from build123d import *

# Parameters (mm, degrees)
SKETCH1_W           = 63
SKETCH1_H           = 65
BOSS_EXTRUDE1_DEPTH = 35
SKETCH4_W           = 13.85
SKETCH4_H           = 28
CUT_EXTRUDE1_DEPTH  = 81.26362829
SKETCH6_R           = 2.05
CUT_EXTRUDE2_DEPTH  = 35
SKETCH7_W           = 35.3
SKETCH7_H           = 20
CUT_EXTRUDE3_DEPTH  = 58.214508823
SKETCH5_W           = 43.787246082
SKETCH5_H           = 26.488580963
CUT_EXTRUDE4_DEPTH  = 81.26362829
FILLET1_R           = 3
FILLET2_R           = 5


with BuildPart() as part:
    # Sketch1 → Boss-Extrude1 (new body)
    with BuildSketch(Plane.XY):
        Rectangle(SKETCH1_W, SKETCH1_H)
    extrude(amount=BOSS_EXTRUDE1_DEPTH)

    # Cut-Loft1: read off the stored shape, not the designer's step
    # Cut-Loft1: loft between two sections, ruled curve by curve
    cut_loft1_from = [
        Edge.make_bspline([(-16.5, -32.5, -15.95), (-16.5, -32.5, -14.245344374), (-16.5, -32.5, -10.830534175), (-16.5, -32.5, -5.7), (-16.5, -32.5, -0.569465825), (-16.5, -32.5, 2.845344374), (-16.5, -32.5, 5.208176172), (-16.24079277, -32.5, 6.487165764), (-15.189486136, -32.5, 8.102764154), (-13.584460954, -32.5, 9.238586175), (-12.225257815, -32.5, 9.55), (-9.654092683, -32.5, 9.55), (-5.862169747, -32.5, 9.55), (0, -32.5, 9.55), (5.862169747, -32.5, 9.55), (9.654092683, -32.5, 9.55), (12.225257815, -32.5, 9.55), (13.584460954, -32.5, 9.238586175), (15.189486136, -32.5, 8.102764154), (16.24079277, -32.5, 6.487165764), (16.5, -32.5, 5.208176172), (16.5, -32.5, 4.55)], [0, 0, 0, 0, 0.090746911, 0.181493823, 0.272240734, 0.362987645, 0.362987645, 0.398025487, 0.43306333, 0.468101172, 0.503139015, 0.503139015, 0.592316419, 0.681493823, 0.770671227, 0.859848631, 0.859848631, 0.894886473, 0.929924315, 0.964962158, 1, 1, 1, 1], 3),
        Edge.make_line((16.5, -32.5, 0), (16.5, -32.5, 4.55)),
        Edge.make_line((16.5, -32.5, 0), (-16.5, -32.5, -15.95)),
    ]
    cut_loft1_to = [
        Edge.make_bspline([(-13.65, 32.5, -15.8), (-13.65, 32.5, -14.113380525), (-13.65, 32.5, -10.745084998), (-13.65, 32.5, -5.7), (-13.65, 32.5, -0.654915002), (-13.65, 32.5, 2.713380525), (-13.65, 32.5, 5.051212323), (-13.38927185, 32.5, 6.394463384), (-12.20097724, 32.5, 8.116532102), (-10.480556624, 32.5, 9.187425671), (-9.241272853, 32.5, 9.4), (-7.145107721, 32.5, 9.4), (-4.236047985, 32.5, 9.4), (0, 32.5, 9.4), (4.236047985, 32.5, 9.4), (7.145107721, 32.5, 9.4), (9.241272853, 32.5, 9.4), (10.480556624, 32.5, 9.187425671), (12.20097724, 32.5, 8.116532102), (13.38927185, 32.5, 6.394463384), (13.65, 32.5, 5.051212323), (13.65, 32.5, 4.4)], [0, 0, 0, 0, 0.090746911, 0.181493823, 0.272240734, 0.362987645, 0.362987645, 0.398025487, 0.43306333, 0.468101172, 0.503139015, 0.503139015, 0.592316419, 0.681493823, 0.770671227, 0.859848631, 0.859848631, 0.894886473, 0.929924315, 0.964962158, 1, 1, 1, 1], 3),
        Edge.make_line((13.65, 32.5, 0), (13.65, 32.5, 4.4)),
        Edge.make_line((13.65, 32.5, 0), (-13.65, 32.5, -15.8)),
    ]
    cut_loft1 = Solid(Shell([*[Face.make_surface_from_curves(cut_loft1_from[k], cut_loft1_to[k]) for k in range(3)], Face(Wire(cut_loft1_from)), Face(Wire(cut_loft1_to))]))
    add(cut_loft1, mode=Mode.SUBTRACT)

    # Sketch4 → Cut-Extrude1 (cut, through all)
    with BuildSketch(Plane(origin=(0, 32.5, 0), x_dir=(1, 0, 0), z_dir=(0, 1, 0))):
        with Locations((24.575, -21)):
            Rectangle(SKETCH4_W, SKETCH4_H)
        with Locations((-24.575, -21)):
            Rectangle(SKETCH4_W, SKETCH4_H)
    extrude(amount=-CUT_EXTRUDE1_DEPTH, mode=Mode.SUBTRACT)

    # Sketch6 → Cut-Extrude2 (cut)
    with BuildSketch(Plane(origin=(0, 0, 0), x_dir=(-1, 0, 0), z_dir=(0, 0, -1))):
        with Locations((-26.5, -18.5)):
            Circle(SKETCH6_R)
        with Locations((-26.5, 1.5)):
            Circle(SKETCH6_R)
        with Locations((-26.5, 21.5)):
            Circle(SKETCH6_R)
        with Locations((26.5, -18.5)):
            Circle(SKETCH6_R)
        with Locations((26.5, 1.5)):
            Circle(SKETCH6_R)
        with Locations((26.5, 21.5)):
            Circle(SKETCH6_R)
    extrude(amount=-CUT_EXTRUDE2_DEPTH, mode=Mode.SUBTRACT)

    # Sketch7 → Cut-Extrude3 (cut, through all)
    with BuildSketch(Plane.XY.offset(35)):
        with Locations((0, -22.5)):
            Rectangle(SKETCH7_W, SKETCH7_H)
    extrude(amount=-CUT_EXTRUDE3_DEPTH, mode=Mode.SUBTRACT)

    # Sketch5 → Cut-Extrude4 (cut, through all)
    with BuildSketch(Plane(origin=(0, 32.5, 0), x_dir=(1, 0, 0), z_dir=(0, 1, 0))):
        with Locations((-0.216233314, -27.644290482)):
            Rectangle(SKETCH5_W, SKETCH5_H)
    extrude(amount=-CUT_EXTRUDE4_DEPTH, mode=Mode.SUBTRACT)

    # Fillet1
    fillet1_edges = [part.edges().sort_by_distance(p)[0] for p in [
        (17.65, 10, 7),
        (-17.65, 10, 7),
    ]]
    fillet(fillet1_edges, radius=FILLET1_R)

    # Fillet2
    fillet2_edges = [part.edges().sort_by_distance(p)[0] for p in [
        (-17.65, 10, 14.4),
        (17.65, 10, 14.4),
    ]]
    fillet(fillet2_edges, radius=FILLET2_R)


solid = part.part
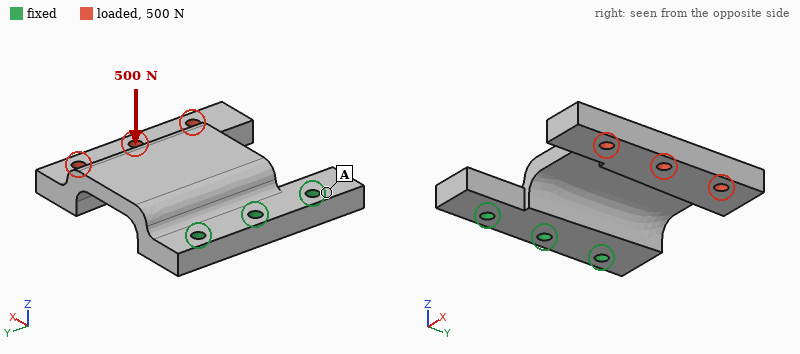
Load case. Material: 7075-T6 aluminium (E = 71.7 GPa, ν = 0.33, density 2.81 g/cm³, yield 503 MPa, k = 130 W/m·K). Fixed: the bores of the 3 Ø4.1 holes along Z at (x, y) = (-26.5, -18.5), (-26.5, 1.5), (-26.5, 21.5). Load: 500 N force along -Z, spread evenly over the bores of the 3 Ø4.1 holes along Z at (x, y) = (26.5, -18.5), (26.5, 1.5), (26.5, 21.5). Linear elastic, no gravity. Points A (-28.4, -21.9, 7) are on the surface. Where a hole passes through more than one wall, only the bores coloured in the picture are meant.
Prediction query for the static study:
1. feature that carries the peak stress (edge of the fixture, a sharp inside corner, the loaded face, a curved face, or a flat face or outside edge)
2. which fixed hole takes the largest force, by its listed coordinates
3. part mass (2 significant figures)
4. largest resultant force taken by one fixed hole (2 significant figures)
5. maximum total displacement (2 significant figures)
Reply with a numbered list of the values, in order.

1. a curved face
2. (-26.5, 1.5)
3. 64 g
4. 390 N
5. 0.88 mm
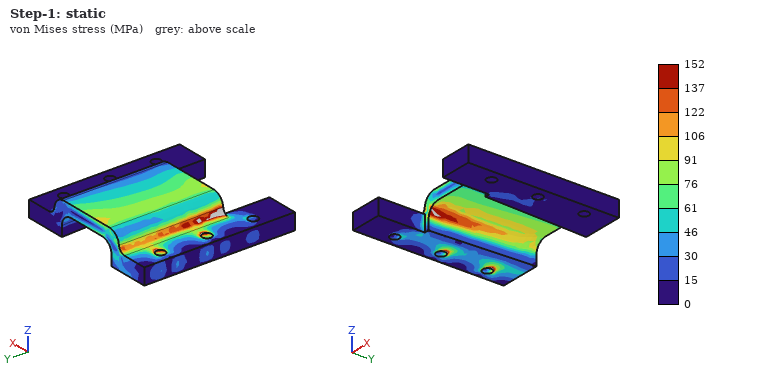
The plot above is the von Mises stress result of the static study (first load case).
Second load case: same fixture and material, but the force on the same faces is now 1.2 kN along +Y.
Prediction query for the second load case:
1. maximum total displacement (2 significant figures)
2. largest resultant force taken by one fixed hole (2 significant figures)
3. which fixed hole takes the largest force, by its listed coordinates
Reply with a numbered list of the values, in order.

1. 0.36 mm
2. 2.2 kN
3. (-26.5, 21.5)
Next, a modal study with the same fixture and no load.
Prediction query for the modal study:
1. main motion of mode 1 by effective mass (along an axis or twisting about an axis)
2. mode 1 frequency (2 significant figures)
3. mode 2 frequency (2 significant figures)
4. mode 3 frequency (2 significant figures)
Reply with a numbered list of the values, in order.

1. along Z
2. 960 Hz
3. 2000 Hz
4. 3600 Hz
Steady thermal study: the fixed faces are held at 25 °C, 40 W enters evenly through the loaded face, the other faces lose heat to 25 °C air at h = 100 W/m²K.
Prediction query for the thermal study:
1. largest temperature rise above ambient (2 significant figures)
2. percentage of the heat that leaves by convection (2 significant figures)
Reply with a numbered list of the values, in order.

1. 53 K
2. 52 %
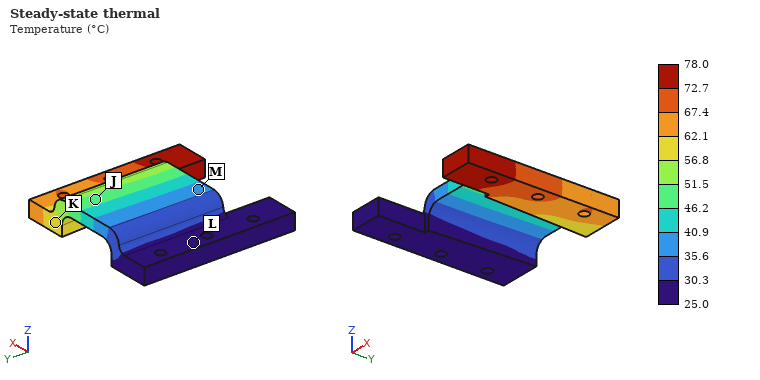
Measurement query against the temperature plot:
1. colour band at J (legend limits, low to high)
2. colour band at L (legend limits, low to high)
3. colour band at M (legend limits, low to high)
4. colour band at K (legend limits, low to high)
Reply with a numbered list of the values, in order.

1. 46.2 to 51.5 °C
2. 25.0 to 30.3 °C
3. 35.6 to 40.9 °C
4. 56.8 to 62.1 °C
